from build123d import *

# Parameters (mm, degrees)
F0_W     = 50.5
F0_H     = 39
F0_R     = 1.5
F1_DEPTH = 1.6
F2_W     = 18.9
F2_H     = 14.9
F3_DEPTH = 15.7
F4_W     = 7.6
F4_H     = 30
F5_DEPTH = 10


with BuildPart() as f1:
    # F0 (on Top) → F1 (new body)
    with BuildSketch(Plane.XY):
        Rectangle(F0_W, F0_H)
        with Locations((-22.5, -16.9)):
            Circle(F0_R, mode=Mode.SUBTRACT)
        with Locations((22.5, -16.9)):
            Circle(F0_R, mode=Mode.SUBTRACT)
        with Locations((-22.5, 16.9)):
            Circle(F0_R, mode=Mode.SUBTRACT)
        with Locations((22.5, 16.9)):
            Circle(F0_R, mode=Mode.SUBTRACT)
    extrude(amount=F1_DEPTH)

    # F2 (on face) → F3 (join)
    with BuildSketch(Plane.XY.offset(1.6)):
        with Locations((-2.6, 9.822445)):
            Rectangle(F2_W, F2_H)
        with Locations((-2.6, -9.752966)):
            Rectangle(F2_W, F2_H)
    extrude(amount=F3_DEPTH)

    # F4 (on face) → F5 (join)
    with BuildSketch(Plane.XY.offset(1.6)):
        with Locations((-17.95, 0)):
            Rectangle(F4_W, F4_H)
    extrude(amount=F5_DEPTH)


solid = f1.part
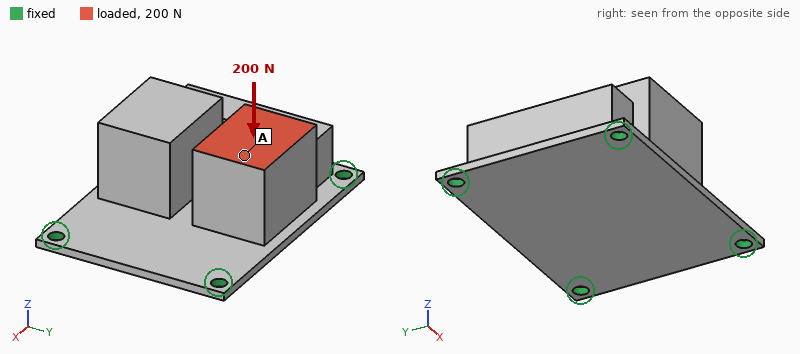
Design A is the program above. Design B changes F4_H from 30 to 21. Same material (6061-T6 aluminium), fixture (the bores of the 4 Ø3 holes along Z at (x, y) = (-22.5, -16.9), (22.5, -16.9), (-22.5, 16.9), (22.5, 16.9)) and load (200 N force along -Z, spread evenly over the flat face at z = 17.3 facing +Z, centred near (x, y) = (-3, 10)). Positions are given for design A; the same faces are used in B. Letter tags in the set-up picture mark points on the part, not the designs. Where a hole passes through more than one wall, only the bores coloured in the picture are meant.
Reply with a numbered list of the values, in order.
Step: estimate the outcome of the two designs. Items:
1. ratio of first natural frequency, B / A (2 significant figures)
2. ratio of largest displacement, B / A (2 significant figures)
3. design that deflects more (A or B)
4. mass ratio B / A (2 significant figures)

1. 0.96
2. 1.1
3. B
4. 0.95
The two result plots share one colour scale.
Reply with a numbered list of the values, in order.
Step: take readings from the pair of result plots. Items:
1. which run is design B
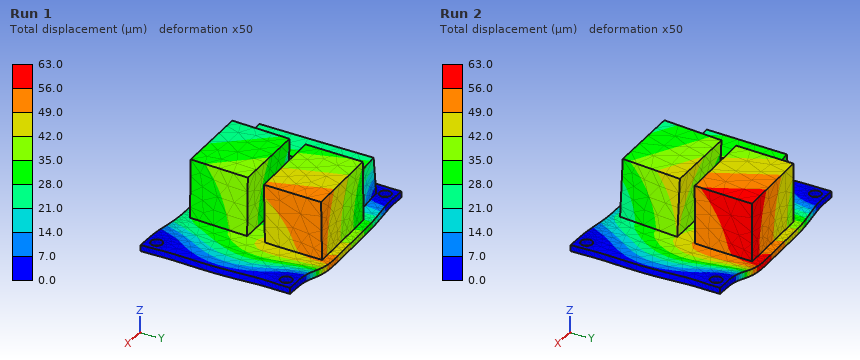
1. Run 2
